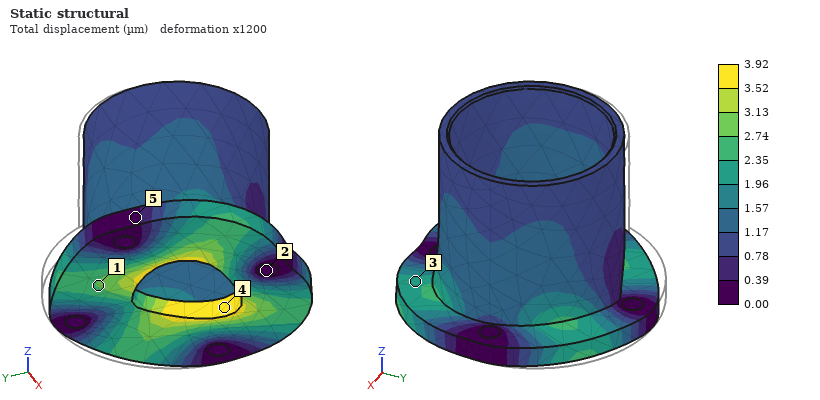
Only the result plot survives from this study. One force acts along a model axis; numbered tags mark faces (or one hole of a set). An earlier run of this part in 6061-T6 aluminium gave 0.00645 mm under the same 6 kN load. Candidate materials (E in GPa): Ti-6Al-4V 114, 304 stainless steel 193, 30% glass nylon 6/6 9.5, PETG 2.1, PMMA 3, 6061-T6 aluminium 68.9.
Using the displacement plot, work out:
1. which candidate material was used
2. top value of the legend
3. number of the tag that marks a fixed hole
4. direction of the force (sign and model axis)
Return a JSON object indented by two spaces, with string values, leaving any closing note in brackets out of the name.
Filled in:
{
  "which candidate material was used": "Ti-6Al-4V",
  "top value of the legend": "3.92 µm",
  "number of the tag that marks a fixed hole": "2",
  "direction of the force": "-Y"
}
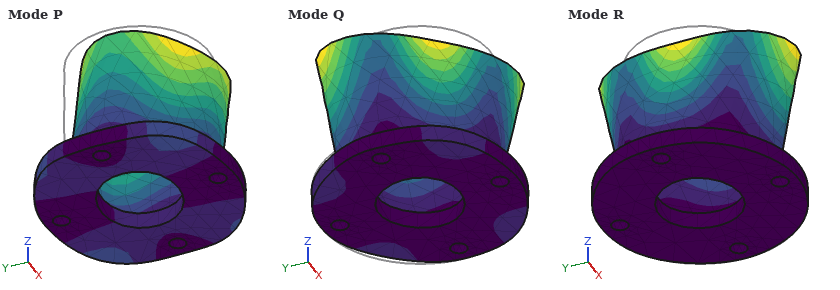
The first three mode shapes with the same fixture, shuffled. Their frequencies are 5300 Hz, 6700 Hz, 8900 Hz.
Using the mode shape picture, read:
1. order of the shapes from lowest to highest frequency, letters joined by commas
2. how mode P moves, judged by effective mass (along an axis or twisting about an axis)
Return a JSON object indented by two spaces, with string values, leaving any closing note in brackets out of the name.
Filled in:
{
  "order of the shapes from lowest to highest frequency, letters joined by commas": "Q, R, P",
  "how mode P moves, judged by effective mass": "along X"
}
